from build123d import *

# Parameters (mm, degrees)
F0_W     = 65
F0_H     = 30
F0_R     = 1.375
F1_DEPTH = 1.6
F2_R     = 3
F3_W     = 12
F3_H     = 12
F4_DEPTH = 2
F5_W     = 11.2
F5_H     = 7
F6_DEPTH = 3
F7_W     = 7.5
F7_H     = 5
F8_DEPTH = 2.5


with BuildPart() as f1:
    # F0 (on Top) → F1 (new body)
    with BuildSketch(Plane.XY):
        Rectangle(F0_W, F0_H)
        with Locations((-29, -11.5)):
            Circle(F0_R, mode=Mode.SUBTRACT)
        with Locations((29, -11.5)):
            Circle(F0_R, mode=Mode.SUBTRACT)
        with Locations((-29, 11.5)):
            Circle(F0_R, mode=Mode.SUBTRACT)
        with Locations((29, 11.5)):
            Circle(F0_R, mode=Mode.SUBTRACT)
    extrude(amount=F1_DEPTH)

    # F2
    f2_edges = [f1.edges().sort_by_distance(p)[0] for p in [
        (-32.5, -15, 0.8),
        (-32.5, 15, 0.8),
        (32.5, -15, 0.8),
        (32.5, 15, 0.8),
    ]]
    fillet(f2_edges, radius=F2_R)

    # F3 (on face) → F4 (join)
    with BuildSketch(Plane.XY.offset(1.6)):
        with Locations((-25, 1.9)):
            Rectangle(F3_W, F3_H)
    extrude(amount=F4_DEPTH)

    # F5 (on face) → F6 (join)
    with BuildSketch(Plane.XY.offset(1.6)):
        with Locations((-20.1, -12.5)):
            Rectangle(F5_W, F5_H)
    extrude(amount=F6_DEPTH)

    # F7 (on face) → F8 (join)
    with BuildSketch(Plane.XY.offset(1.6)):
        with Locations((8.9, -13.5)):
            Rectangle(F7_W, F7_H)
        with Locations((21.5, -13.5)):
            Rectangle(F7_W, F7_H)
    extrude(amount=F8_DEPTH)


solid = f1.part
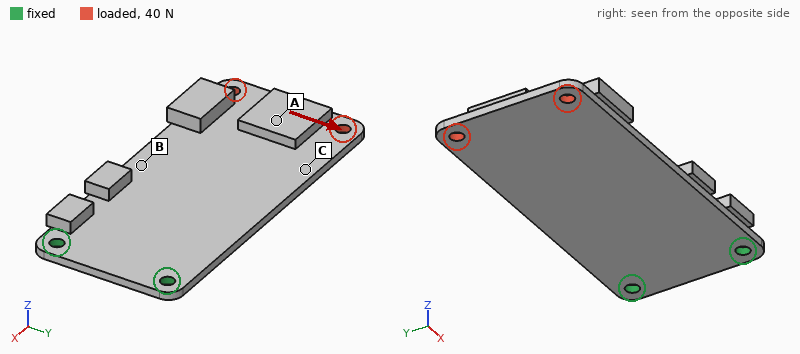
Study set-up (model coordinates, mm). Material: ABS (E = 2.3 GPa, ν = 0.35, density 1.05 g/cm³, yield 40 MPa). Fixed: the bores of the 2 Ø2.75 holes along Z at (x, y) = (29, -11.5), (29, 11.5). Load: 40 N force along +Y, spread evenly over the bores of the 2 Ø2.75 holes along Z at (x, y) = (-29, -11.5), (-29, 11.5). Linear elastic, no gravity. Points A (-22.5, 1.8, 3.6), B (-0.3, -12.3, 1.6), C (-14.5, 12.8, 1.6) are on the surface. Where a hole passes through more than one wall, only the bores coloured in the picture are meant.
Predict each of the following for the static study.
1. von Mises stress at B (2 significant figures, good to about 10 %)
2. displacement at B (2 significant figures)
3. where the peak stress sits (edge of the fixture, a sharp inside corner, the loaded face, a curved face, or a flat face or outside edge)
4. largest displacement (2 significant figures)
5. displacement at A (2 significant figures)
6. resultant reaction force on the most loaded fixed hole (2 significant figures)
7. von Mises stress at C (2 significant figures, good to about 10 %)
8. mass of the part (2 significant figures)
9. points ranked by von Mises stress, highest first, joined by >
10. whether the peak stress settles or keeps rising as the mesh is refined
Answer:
4.4 MPa
0.18 mm
edge of the fixture
0.51 mm
0.38 mm
100 N
2.4 MPa
4.0 g
B > C > A
keeps rising
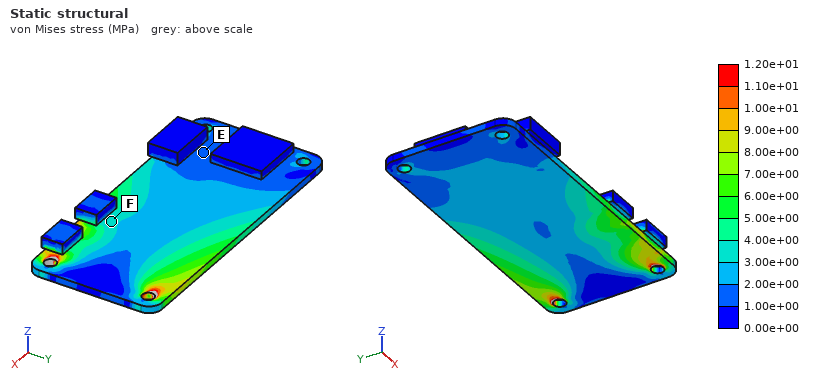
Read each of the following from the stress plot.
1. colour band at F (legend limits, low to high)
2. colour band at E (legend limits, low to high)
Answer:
3.00e+00 to 4.00e+00 MPa
1.00e+00 to 2.00e+00 MPa
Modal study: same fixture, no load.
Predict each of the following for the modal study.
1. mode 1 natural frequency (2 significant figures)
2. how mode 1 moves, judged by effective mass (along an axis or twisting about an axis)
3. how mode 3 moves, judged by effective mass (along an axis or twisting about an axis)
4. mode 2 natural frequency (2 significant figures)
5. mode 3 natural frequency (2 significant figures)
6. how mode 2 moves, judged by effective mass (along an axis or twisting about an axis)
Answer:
90 Hz
along Z
along Z
420 Hz
620 Hz
twisting about X
